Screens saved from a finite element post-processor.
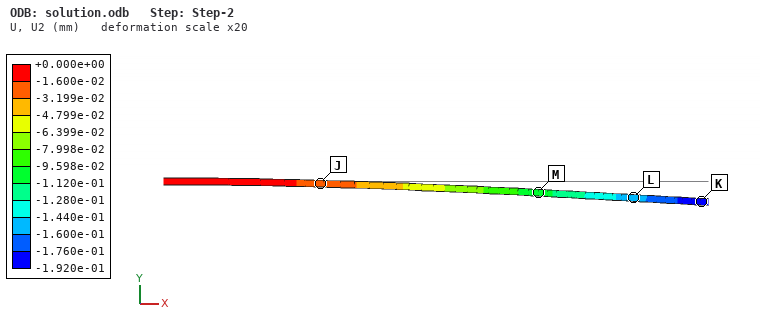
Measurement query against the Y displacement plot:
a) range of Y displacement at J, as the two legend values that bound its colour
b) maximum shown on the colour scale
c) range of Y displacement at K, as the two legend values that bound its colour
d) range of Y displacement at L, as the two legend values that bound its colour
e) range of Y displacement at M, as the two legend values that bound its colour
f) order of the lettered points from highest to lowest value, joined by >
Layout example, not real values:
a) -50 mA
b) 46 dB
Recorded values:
a) -3.199e-02 to -1.600e-02 mm
b) +0.000e+00 mm
c) -1.920e-01 to -1.760e-01 mm
d) -1.600e-01 to -1.440e-01 mm
e) -1.120e-01 to -9.598e-02 mm
f) J > M > L > K
